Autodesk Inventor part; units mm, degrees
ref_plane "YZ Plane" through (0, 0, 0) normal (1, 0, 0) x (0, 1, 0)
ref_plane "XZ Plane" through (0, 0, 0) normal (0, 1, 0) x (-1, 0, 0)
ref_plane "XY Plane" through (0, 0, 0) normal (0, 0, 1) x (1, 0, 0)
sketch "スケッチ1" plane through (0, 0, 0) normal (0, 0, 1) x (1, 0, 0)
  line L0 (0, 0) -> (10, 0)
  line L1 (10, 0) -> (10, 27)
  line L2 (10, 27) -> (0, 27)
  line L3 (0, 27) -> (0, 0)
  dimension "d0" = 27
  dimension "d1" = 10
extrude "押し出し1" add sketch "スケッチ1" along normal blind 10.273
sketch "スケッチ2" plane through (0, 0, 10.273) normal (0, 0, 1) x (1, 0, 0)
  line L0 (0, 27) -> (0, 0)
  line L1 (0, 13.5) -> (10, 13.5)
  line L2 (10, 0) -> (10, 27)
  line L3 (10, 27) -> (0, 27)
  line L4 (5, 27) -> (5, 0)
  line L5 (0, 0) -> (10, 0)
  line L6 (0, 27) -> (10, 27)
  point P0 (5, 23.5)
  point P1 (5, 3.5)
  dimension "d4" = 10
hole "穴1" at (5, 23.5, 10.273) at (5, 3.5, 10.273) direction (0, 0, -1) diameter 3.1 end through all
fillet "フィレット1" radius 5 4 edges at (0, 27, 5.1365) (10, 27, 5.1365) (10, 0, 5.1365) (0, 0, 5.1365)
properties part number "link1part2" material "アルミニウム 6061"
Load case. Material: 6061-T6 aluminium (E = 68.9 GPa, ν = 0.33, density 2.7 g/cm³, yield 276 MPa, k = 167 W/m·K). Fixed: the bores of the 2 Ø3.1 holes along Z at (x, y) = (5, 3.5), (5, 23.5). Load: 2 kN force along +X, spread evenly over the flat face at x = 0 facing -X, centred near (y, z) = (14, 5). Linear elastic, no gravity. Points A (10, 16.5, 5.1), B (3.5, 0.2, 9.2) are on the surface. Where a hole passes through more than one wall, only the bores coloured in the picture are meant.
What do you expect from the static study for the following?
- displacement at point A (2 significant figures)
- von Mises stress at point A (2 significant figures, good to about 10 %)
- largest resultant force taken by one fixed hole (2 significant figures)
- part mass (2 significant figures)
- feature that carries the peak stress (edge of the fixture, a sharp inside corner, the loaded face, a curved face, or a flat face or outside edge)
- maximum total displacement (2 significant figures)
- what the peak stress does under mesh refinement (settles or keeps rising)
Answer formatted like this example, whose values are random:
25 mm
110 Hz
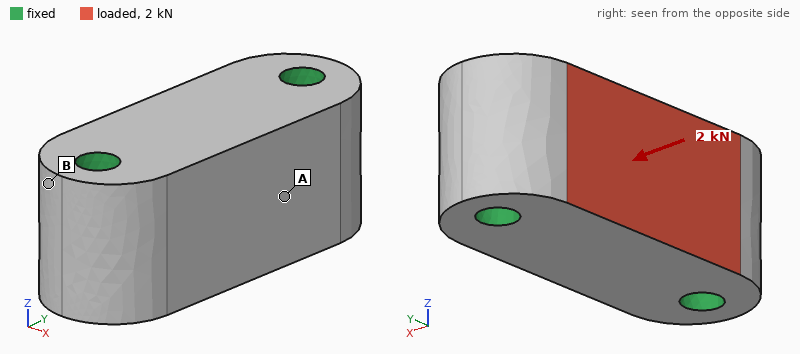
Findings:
2.9 µm
16 MPa
1.0 kN
6.5 g
edge of the fixture
4.4 µm
keeps rising
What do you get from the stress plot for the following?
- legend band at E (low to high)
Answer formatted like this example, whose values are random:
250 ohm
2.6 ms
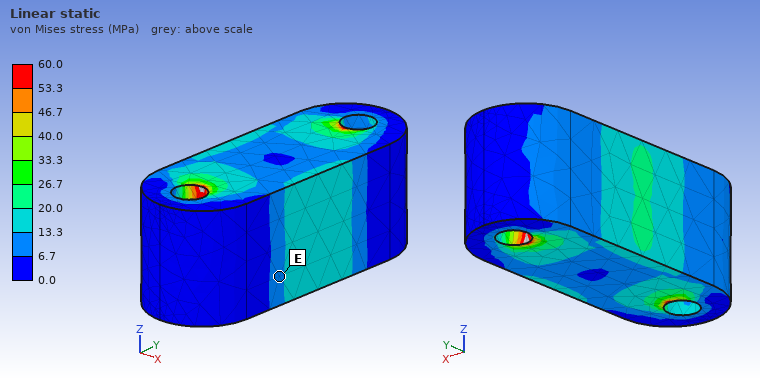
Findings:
6.7 to 13.3 MPa
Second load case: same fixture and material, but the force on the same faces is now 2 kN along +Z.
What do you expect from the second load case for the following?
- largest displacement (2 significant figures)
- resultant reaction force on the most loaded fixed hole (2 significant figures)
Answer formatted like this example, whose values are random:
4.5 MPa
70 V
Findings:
9.7 µm
1.0 kN
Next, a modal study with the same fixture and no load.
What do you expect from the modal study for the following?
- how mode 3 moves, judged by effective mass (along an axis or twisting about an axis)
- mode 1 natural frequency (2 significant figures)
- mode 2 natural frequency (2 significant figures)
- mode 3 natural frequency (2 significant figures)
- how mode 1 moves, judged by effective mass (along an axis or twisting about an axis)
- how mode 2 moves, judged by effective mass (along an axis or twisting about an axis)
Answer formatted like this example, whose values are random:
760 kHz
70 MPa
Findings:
twisting about Y
58 kHz
65 kHz
72 kHz
along X
along Z
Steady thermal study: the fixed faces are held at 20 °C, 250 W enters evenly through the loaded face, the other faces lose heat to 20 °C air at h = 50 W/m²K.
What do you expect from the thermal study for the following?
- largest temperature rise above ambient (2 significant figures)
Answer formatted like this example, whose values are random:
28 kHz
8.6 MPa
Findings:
68 K
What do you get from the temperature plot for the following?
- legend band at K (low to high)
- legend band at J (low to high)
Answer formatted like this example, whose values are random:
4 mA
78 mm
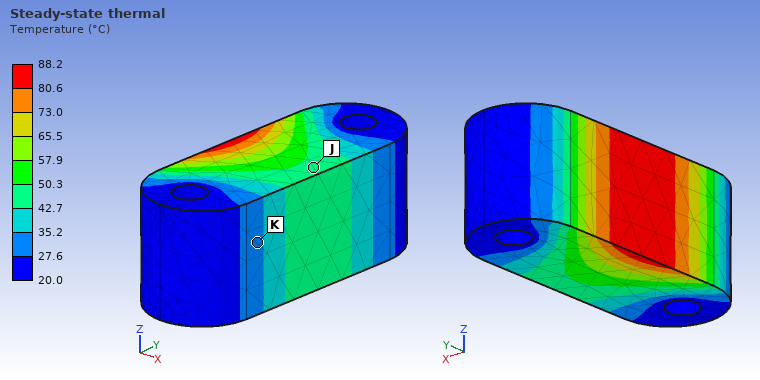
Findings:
27.6 to 35.2 °C
42.7 to 50.3 °C
